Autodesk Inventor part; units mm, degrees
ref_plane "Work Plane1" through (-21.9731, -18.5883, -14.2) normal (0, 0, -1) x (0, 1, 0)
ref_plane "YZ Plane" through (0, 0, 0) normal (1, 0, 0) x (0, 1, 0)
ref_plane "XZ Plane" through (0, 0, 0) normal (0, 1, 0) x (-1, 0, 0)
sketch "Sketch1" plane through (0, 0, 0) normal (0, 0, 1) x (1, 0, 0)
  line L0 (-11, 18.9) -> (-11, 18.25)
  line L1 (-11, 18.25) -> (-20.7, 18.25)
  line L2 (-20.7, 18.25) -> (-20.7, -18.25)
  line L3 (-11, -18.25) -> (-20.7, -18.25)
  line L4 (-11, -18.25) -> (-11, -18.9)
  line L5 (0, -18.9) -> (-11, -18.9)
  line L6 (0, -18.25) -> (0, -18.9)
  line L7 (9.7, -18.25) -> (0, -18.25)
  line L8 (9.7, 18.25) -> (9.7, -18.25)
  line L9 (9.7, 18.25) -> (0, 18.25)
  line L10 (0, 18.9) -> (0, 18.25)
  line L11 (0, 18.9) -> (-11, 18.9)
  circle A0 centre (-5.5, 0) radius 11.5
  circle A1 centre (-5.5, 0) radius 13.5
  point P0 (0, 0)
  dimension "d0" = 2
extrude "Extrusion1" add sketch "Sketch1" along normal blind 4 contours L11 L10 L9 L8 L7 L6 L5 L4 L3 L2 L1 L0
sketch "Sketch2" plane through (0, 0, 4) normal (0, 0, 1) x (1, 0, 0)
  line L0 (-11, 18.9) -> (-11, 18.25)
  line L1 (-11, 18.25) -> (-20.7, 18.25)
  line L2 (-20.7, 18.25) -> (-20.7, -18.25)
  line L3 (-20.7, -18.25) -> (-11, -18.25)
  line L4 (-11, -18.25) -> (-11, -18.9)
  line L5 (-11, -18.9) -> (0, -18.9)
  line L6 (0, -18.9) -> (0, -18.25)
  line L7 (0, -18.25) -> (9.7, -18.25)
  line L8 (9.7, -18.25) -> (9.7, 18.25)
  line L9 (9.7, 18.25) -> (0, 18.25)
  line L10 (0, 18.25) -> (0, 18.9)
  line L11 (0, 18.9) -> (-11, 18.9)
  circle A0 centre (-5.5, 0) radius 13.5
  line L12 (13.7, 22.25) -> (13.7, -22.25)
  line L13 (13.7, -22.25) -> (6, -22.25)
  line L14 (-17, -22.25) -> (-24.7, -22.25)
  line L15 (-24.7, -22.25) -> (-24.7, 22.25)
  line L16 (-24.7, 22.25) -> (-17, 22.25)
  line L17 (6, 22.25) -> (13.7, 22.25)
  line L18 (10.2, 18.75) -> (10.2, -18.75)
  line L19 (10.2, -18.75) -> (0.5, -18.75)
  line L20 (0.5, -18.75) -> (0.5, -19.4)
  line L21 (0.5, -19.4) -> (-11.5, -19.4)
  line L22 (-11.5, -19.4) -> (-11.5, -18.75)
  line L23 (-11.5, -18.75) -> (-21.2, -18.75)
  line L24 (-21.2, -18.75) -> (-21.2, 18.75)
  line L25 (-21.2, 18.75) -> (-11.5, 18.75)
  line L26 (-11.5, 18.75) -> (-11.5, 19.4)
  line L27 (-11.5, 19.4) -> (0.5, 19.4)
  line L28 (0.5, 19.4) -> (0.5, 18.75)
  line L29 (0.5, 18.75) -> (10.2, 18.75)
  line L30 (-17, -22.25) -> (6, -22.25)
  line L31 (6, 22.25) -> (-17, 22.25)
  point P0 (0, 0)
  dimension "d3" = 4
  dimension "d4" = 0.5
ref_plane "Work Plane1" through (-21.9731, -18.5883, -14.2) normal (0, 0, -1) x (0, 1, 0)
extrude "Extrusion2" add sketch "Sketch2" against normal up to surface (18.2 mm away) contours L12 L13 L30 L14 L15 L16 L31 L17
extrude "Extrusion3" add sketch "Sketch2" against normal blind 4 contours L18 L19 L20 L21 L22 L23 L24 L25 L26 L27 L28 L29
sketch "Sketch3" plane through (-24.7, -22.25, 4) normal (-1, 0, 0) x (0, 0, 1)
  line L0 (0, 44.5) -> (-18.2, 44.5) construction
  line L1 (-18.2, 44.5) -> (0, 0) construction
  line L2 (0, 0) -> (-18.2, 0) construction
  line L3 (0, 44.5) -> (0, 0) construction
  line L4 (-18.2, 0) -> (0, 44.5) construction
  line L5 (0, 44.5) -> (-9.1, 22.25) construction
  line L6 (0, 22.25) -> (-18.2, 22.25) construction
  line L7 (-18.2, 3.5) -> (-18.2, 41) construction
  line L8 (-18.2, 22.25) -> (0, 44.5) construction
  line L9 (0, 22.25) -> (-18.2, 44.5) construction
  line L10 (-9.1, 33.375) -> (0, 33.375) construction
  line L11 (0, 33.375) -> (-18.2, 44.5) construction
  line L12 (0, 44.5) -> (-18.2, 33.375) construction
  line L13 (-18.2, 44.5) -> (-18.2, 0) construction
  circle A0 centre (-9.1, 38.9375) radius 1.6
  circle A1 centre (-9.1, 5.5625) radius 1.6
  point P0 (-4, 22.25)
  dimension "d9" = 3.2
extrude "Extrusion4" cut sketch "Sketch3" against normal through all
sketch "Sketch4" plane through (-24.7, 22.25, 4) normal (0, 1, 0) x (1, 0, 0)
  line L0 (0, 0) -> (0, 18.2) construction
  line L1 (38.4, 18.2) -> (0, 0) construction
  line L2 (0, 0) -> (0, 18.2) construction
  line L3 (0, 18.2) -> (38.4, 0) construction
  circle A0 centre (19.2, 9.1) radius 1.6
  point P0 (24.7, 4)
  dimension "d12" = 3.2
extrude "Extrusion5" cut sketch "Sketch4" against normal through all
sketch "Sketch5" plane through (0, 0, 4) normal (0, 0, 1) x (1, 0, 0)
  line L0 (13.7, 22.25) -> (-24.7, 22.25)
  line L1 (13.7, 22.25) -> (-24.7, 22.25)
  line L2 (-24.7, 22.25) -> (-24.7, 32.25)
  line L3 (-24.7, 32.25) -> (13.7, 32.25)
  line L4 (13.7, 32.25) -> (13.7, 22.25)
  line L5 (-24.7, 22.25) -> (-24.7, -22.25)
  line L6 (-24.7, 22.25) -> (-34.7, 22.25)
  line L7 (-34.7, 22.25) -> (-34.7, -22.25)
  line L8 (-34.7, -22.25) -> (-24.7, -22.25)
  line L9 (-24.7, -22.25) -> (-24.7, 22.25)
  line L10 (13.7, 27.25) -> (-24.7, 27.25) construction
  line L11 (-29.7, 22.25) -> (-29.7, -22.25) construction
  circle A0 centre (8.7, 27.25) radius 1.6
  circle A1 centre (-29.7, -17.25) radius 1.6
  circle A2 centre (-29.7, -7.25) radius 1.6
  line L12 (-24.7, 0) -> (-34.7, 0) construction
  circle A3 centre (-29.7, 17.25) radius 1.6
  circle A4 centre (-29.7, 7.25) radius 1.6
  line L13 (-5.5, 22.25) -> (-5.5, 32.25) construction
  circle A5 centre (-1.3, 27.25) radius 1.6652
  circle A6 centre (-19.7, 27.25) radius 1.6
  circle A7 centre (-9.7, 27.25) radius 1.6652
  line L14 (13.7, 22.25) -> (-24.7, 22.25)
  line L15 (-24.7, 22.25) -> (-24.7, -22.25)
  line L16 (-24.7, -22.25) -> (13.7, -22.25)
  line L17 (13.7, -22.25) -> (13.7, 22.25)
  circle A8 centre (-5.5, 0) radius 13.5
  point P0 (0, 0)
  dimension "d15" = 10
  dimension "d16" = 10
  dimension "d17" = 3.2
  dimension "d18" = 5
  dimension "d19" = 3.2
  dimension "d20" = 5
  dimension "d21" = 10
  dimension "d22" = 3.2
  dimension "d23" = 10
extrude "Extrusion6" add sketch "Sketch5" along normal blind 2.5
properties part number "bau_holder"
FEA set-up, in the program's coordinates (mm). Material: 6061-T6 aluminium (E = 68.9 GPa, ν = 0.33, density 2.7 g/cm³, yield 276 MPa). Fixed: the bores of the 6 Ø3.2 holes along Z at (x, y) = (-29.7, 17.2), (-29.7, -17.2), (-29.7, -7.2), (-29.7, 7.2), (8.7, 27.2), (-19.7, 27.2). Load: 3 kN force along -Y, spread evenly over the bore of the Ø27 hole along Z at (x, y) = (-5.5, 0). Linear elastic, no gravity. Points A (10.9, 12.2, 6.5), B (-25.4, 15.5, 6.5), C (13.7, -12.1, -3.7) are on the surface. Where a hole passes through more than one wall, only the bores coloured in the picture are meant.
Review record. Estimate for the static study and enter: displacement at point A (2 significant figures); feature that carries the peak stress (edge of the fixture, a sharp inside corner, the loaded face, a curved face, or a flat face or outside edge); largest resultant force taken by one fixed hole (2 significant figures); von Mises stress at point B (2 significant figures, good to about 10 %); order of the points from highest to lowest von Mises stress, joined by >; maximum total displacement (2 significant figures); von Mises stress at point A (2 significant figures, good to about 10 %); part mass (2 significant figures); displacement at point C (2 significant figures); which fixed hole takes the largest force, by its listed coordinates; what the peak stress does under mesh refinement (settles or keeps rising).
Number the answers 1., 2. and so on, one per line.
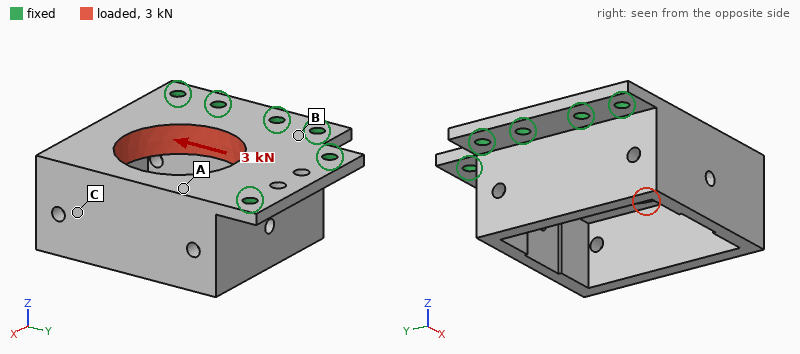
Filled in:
1. 18 µm
2. edge of the fixture
3. 1.2 kN
4. 9.9 MPa
5. A > B > C
6. 50 µm
7. 26 MPa
8. 44 g
9. 40 µm
10. (8.7, 27.2)
11. keeps rising
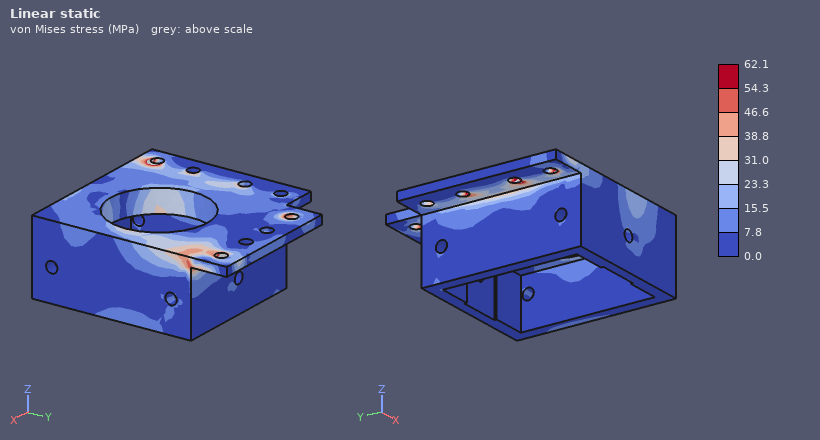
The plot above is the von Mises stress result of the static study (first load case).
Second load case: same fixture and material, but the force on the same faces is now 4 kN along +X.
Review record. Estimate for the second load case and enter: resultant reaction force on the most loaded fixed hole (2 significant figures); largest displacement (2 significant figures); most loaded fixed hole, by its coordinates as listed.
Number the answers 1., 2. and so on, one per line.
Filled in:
1. 1.2 kN
2. 90 µm
3. (-29.7, -17.2)
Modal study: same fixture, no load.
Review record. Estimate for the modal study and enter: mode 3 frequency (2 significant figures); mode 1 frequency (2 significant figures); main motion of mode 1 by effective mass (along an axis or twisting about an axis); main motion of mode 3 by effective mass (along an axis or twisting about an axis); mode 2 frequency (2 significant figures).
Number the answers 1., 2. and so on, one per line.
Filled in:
1. 11 kHz
2. 2000 Hz
3. along Z
4. along Z
5. 9800 Hz
